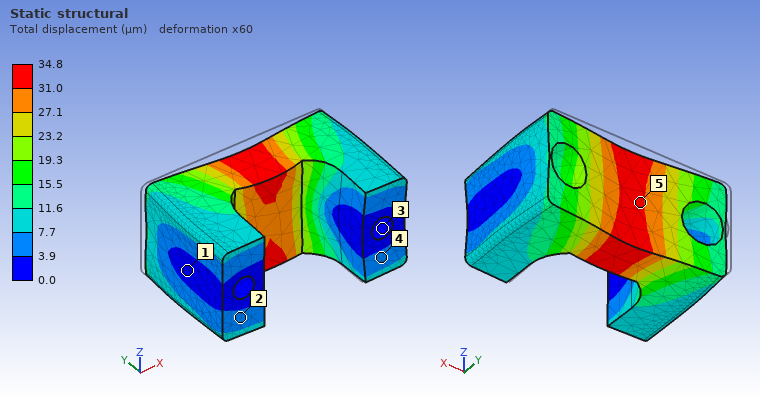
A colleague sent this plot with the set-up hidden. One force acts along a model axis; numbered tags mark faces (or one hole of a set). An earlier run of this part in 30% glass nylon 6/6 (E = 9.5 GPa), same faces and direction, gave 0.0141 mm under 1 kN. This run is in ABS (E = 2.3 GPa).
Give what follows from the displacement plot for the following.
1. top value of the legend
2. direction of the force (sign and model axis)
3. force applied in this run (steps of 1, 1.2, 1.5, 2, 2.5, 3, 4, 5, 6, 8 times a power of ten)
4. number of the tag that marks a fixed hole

34.8 µm
-Y
600 N
3
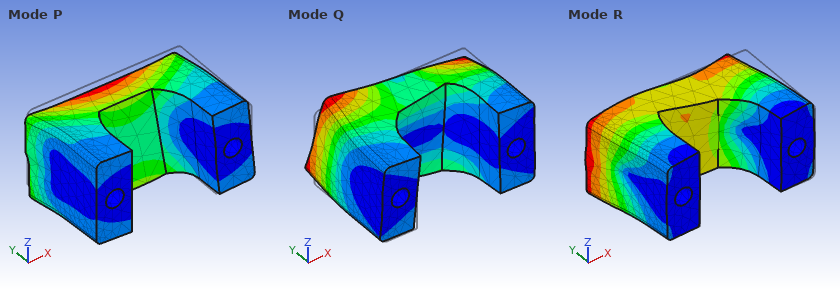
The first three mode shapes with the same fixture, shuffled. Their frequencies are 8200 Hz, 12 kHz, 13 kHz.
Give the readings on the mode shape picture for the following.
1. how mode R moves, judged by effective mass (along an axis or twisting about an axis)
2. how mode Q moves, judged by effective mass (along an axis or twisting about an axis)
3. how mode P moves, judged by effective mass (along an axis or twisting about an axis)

along X
twisting about Y
along Z
